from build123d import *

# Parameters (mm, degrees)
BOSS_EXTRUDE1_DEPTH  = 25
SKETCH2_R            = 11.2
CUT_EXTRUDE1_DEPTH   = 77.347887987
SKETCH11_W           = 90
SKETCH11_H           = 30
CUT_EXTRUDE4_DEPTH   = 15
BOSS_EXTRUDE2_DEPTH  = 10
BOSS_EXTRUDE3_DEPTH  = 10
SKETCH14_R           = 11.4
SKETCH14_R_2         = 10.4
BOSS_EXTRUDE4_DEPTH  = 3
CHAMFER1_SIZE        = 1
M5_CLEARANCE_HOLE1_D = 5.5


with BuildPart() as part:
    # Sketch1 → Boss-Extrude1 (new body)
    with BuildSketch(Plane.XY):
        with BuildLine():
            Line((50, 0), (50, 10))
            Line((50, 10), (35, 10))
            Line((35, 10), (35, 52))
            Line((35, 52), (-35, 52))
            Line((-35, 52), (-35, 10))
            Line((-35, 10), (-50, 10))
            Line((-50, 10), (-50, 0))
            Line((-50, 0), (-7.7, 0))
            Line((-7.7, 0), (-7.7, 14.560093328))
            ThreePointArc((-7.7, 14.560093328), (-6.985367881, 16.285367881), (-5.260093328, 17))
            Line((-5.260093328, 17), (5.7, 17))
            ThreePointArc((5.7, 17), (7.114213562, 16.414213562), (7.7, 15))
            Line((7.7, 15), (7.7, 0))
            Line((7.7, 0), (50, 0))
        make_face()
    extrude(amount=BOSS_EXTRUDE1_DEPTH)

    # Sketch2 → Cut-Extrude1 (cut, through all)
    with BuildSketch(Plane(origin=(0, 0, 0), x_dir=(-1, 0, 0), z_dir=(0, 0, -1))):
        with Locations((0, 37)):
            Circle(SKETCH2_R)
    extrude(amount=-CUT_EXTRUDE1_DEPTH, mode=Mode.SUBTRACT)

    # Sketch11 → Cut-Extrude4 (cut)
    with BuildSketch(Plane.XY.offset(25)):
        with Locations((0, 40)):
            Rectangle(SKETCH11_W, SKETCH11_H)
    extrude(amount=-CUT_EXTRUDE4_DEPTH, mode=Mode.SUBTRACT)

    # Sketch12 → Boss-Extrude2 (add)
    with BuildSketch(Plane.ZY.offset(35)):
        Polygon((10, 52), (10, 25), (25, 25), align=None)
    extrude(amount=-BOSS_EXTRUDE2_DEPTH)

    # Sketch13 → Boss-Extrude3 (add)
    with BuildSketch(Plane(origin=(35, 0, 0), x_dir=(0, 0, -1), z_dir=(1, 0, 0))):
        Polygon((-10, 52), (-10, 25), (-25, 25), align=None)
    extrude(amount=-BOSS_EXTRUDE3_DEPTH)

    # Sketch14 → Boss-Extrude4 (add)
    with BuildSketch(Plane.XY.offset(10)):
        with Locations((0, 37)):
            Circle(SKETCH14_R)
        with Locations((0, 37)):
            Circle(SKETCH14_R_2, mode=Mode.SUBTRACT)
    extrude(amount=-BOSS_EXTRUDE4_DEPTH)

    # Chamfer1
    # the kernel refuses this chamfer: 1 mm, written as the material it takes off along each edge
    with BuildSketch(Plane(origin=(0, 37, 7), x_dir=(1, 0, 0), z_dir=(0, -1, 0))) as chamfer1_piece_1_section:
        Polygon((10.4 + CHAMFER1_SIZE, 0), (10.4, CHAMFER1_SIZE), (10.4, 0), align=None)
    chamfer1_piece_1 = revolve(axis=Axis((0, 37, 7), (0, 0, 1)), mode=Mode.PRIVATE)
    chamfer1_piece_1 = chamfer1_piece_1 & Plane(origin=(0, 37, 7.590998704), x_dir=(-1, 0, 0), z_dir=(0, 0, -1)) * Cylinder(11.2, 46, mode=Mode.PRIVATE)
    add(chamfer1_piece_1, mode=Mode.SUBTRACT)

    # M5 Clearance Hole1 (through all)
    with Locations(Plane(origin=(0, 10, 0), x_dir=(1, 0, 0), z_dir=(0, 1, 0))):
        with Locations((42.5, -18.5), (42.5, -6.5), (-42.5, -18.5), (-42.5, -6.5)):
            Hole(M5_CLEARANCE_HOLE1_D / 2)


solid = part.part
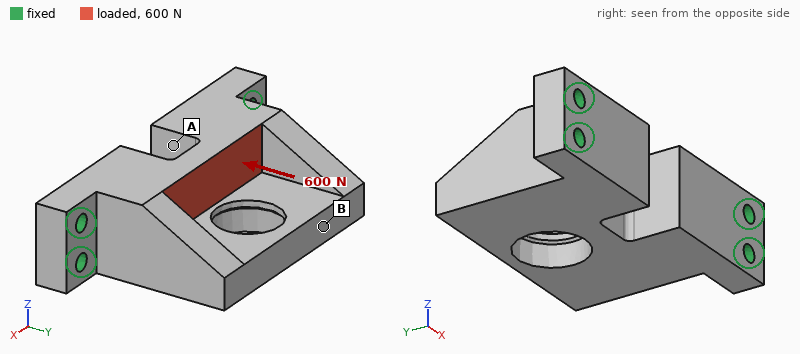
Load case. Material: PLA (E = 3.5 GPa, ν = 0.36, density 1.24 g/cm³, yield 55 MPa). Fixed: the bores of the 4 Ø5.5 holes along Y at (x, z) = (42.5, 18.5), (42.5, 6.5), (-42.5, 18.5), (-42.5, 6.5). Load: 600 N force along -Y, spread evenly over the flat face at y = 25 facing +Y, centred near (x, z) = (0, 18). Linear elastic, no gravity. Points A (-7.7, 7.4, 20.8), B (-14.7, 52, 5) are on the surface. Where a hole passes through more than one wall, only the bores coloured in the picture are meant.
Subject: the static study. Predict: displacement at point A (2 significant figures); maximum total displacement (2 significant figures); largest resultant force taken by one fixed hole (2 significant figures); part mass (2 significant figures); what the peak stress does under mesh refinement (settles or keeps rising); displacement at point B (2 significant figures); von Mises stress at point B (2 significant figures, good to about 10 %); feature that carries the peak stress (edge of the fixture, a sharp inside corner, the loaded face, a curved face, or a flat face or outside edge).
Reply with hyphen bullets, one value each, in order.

- 45 µm
- 66 µm
- 270 N
- 78 g
- keeps rising
- 52 µm
- 1.2 MPa
- edge of the fixture
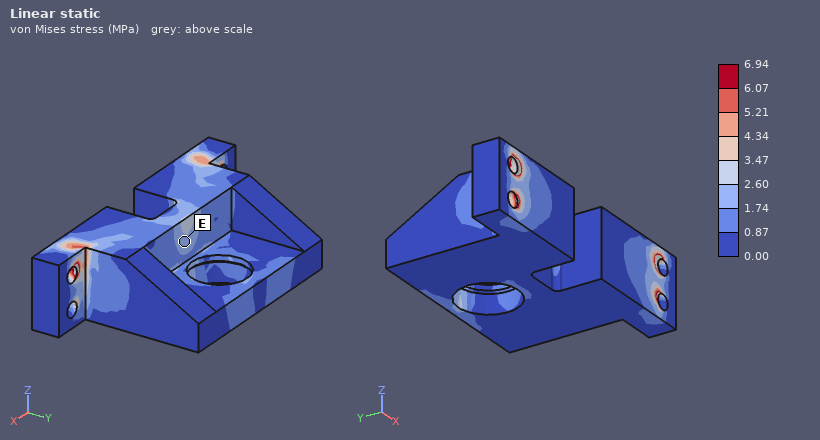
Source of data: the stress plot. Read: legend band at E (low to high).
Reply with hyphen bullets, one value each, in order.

- 1.74 to 2.60 MPa
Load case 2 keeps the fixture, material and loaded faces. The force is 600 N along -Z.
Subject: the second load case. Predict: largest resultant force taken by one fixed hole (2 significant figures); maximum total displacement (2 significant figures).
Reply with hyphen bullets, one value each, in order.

- 490 N
- 0.25 mm
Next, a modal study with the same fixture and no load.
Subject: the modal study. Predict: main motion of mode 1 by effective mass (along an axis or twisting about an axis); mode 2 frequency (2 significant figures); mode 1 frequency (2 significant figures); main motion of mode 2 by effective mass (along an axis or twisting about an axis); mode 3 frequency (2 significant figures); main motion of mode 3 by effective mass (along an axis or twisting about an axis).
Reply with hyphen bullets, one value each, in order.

- along Z
- 2200 Hz
- 1300 Hz
- twisting about Y
- 3200 Hz
- along Y
